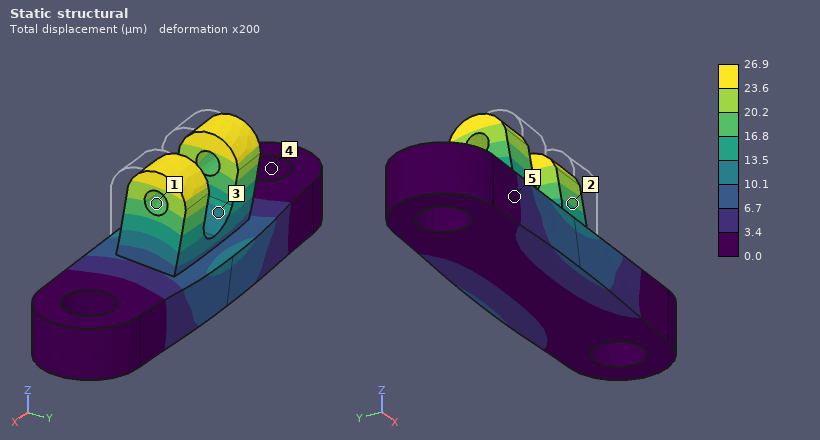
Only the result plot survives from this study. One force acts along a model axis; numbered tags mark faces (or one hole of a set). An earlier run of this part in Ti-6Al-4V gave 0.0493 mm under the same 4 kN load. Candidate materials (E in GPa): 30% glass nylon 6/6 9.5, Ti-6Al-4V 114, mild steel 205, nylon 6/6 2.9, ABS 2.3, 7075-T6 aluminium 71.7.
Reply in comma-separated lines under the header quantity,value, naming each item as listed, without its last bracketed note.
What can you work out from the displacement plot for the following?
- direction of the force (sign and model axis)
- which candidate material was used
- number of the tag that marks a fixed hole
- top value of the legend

quantity,value
direction of the force,+Y
which candidate material was used,mild steel
number of the tag that marks a fixed hole,4
top value of the legend,26.9 µm
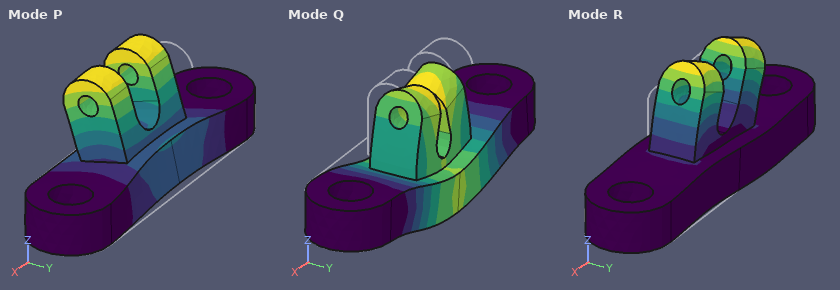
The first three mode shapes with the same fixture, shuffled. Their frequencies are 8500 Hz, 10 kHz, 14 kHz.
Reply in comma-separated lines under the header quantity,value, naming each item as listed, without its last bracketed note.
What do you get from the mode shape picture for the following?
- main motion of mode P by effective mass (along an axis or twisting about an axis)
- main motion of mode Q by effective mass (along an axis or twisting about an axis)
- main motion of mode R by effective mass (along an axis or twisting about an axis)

quantity,value
main motion of mode P by effective mass,along Y
main motion of mode Q by effective mass,along Z
main motion of mode R by effective mass,along X
